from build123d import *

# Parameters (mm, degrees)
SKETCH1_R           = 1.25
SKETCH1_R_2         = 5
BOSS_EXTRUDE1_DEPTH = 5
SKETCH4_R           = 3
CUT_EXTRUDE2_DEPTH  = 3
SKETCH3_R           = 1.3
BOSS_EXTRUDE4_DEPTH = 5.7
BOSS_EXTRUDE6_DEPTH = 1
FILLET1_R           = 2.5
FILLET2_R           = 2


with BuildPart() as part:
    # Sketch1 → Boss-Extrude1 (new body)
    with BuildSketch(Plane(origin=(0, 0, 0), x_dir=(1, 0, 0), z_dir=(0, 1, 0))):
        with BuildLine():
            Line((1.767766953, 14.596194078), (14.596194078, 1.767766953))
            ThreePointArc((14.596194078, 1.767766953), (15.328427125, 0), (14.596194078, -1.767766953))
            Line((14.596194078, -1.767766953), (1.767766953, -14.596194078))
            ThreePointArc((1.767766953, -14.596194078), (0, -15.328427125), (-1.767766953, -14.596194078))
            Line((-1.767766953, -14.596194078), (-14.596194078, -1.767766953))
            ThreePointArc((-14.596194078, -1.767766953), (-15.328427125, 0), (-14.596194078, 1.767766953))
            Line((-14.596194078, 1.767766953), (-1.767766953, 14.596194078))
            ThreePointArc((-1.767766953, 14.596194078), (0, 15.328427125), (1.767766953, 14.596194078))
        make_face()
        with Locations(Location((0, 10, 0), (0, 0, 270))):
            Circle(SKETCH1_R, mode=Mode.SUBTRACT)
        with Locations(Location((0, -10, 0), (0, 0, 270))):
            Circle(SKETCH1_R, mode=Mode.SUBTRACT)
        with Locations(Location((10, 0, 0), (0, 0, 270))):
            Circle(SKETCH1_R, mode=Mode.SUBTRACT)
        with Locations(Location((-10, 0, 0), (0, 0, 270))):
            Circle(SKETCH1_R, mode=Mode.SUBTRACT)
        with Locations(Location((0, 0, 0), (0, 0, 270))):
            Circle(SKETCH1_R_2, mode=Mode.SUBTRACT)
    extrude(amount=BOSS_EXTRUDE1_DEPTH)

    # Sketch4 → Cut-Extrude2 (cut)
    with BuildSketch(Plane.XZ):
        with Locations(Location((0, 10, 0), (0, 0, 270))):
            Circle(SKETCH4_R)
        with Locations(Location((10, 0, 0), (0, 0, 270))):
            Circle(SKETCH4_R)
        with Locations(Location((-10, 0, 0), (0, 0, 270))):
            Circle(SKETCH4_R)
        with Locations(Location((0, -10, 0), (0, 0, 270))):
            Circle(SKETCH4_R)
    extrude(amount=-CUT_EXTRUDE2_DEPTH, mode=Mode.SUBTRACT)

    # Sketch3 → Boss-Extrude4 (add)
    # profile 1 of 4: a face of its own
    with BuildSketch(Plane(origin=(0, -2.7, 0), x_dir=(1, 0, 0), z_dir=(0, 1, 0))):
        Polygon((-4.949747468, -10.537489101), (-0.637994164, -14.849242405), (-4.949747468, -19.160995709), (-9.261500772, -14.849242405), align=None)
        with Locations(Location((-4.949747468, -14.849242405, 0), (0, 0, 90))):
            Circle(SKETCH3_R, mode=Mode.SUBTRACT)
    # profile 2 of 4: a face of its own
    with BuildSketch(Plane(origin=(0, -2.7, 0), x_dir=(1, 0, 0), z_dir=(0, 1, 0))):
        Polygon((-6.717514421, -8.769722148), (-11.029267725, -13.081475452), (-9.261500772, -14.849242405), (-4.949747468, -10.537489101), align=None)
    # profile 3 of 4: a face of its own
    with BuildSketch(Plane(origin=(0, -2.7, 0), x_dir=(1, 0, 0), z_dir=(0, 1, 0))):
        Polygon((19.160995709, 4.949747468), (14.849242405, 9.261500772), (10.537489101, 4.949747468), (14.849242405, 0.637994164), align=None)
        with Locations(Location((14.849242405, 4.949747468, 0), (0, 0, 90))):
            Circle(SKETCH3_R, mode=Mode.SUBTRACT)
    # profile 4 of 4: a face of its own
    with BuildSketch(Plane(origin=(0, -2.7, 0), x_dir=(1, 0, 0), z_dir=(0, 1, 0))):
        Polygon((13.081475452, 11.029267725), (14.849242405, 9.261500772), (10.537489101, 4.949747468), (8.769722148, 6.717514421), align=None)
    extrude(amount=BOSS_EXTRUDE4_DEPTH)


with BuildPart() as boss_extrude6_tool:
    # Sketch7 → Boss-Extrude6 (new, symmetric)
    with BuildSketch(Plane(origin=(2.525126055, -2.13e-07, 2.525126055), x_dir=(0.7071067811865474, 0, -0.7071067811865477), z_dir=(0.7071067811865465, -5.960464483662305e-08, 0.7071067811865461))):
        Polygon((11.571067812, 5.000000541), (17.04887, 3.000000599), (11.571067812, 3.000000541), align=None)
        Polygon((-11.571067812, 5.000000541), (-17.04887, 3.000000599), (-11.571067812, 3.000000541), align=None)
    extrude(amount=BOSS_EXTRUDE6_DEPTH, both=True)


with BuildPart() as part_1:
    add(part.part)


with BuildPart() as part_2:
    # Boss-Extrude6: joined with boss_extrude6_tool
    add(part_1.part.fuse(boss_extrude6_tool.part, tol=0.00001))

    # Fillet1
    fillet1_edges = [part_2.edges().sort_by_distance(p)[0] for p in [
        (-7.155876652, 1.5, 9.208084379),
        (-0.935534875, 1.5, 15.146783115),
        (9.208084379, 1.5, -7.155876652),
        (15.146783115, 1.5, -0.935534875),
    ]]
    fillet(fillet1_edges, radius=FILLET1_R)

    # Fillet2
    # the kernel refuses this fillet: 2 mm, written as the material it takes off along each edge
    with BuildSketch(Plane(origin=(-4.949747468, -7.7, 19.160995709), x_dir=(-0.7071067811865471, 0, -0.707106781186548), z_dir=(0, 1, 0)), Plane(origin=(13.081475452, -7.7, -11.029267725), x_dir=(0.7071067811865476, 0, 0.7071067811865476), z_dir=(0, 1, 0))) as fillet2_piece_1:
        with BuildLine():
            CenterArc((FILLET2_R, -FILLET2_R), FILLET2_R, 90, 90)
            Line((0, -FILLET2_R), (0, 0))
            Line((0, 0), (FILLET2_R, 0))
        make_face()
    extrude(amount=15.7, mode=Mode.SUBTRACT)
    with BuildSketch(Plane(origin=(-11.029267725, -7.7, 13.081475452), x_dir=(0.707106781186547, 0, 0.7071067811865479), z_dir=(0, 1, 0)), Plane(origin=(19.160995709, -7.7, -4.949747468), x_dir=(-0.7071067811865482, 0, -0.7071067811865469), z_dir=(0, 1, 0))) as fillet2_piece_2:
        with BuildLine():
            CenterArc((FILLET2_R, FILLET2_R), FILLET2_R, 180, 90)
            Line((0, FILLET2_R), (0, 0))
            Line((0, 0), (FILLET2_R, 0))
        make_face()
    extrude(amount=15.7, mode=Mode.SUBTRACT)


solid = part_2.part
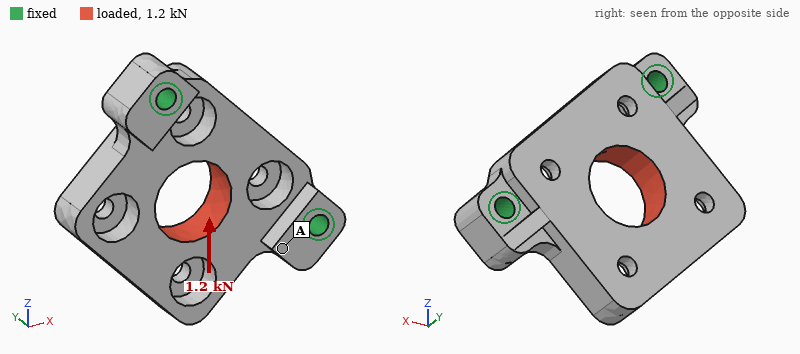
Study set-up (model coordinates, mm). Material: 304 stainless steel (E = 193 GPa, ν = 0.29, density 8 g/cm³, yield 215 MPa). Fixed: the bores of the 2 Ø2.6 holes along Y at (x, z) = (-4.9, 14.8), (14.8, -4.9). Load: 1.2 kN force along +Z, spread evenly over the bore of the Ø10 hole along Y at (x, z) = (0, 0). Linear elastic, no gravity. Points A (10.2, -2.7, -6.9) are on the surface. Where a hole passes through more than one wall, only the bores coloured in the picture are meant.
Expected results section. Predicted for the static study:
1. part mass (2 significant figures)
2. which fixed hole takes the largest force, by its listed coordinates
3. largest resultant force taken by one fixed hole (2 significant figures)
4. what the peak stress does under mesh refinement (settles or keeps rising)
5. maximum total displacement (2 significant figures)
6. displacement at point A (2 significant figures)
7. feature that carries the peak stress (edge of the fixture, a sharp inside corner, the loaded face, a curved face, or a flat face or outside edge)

19 g
(-4.9, 14.8)
790 N
keeps rising
4.7 µm
0.82 µm
edge of the fixture
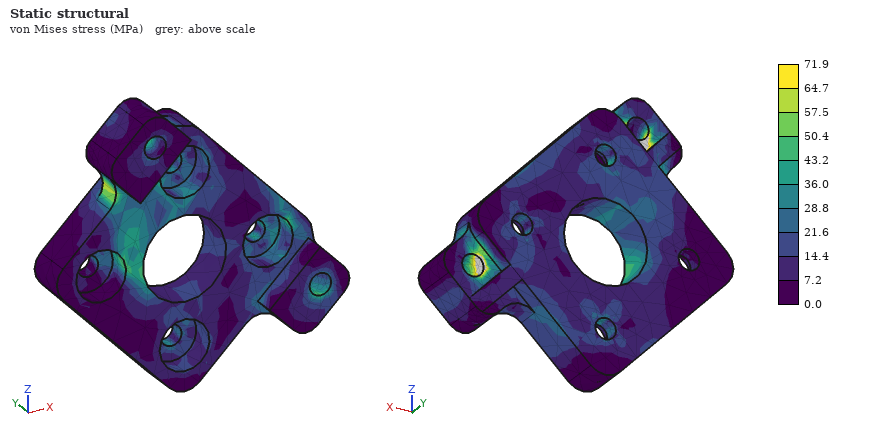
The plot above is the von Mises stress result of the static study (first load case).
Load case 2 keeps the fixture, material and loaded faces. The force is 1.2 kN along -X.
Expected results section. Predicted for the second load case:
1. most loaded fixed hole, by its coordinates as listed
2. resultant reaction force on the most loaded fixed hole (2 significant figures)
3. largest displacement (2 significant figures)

(14.8, -4.9)
790 N
4.7 µm
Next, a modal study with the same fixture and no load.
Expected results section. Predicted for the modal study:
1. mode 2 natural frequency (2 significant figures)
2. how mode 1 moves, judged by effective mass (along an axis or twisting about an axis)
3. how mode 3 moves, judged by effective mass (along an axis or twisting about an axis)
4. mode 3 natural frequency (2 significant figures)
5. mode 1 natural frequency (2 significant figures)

20 kHz
along Y
along Y
25 kHz
8400 Hz
